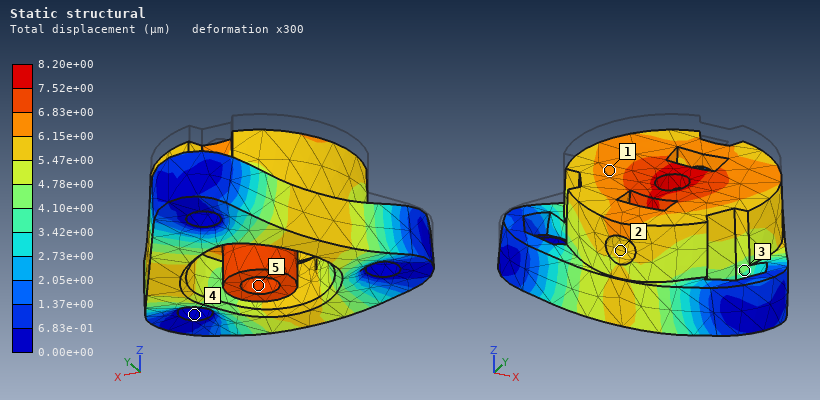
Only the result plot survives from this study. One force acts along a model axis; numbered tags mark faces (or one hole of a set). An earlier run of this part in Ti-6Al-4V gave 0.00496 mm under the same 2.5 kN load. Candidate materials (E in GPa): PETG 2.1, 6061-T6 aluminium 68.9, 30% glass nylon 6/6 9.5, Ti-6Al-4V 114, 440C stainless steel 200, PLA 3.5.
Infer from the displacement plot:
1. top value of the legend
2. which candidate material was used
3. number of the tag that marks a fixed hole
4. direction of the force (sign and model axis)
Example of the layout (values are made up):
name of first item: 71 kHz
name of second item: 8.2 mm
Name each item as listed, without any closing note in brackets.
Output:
top value of the legend: 8.20e+00 µm
which candidate material was used: 6061-T6 aluminium
number of the tag that marks a fixed hole: 4
direction of the force: -Z
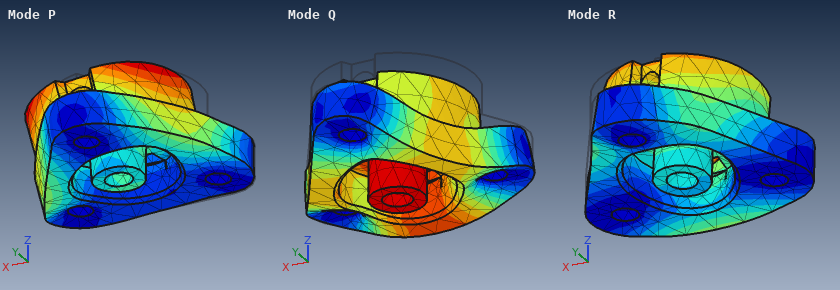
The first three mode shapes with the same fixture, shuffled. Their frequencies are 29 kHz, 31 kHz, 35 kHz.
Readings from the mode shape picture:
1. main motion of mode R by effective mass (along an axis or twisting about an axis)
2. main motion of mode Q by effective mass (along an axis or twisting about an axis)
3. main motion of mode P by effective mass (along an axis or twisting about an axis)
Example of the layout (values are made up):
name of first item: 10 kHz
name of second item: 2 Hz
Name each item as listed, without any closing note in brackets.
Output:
main motion of mode R by effective mass: along Y
main motion of mode Q by effective mass: along Z
main motion of mode P by effective mass: along X
